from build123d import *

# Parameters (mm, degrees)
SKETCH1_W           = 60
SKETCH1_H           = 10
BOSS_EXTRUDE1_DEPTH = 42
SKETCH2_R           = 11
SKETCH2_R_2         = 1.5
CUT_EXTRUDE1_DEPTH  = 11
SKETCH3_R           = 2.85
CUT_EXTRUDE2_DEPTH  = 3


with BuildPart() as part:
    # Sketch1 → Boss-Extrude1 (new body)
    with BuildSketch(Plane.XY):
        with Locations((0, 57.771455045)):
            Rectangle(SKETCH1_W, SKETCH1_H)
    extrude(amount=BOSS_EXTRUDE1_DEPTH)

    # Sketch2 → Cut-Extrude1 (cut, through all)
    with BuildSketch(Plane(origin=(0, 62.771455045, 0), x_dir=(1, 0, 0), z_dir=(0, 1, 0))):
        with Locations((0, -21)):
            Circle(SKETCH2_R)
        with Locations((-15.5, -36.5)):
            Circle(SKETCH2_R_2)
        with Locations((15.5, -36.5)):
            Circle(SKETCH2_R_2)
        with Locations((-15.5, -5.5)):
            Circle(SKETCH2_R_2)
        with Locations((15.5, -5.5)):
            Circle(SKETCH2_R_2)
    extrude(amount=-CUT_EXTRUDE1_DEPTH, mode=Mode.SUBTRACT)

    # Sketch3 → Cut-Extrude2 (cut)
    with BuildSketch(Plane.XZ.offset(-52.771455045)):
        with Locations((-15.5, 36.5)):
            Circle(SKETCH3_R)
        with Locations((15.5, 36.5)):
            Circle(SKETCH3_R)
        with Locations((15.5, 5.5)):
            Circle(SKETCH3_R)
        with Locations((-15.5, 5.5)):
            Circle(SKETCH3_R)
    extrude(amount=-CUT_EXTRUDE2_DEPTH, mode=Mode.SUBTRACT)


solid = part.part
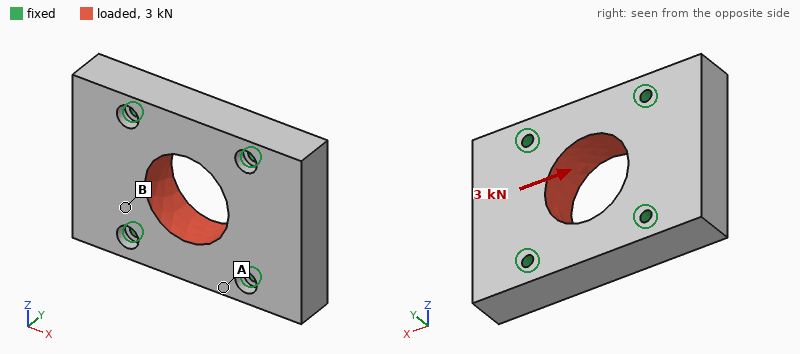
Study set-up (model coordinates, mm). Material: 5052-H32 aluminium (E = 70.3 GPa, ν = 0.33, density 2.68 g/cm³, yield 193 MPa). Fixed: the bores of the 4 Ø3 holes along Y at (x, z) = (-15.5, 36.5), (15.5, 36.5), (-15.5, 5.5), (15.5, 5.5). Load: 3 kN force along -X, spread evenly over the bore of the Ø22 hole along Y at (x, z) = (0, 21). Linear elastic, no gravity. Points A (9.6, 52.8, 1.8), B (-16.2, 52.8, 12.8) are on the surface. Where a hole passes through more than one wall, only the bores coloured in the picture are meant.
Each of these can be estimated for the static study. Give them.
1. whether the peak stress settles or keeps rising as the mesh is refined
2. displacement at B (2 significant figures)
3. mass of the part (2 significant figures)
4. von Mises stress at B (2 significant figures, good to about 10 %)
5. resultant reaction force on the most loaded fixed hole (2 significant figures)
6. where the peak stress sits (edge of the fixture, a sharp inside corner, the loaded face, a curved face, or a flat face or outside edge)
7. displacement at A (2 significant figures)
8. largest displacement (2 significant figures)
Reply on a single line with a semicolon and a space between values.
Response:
keeps rising; 1.5 µm; 56 g; 4.2 MPa; 750 N; edge of the fixture; 0.61 µm; 2.3 µm
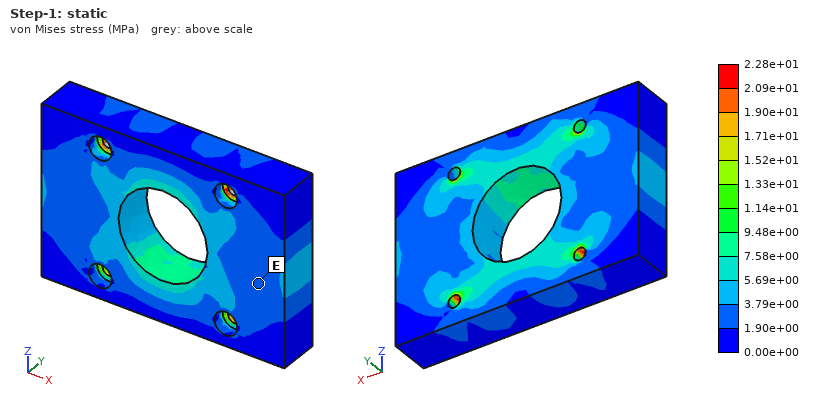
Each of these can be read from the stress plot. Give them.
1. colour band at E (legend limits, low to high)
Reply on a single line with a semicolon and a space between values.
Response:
1.90e+00 to 3.79e+00 MPa
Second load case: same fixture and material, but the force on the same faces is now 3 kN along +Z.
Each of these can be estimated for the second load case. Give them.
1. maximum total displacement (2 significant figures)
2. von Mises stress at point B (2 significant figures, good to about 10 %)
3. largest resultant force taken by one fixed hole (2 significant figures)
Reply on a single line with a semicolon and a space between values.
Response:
3.2 µm; 4.0 MPa; 780 N
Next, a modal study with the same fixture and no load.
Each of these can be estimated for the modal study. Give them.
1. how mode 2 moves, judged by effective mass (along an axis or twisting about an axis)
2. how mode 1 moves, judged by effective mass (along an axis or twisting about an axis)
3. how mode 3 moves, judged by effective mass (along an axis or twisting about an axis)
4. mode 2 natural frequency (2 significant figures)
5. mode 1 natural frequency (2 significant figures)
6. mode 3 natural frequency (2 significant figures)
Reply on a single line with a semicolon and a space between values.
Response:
twisting about Z; along Y; along Y; 18 kHz; 17 kHz; 27 kHz
